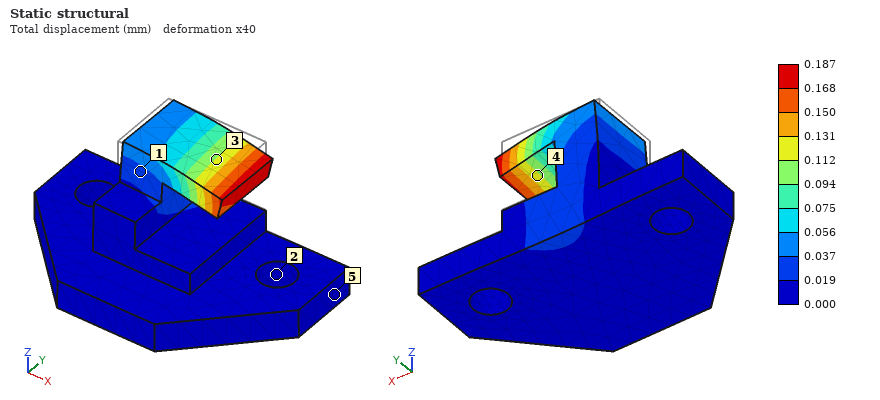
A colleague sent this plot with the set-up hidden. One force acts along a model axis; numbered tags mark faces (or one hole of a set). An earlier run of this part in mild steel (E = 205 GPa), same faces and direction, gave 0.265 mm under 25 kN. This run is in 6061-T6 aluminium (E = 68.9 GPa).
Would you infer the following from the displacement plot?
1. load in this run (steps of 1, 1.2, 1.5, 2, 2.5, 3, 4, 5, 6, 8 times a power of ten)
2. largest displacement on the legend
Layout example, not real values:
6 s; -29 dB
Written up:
6 kN; 0.187 mm
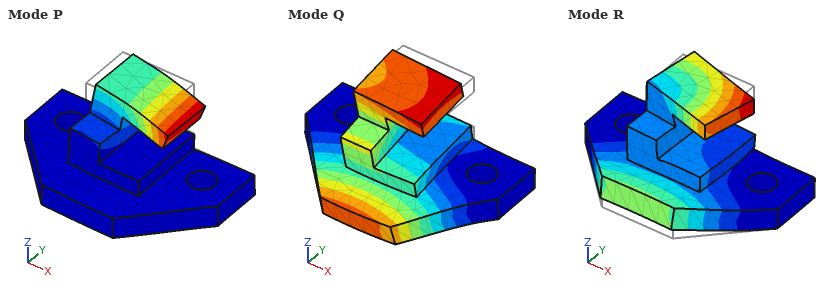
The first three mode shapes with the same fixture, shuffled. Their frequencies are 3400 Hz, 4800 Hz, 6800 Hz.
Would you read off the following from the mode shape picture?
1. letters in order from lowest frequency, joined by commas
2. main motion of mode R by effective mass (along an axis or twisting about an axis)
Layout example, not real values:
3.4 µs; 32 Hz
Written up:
Q, P, R; along Z
